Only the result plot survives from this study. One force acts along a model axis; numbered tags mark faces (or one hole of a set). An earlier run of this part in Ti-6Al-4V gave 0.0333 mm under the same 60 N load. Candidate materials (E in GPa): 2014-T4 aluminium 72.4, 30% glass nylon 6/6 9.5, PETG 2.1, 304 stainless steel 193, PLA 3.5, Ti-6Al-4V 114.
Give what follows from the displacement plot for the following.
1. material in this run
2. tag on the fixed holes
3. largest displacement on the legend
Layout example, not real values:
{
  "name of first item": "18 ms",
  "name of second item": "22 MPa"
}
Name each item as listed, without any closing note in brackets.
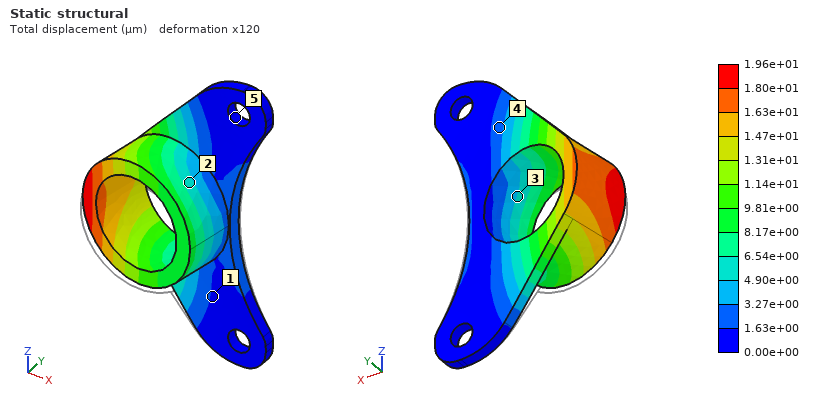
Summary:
{
  "material in this run": "304 stainless steel",
  "tag on the fixed holes": "5",
  "largest displacement on the legend": "1.96e+01 µm"
}
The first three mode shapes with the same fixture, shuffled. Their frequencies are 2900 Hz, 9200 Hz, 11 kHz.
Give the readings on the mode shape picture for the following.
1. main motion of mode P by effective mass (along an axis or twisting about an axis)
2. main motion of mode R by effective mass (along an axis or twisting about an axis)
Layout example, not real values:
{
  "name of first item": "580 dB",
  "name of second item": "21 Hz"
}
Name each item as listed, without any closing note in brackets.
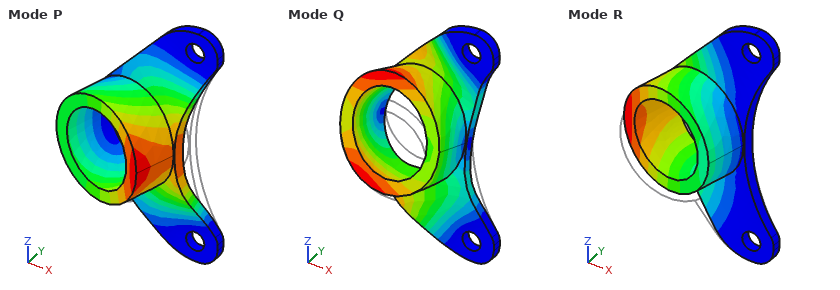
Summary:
{
  "main motion of mode P by effective mass": "along Y",
  "main motion of mode R by effective mass": "along Y"
}
